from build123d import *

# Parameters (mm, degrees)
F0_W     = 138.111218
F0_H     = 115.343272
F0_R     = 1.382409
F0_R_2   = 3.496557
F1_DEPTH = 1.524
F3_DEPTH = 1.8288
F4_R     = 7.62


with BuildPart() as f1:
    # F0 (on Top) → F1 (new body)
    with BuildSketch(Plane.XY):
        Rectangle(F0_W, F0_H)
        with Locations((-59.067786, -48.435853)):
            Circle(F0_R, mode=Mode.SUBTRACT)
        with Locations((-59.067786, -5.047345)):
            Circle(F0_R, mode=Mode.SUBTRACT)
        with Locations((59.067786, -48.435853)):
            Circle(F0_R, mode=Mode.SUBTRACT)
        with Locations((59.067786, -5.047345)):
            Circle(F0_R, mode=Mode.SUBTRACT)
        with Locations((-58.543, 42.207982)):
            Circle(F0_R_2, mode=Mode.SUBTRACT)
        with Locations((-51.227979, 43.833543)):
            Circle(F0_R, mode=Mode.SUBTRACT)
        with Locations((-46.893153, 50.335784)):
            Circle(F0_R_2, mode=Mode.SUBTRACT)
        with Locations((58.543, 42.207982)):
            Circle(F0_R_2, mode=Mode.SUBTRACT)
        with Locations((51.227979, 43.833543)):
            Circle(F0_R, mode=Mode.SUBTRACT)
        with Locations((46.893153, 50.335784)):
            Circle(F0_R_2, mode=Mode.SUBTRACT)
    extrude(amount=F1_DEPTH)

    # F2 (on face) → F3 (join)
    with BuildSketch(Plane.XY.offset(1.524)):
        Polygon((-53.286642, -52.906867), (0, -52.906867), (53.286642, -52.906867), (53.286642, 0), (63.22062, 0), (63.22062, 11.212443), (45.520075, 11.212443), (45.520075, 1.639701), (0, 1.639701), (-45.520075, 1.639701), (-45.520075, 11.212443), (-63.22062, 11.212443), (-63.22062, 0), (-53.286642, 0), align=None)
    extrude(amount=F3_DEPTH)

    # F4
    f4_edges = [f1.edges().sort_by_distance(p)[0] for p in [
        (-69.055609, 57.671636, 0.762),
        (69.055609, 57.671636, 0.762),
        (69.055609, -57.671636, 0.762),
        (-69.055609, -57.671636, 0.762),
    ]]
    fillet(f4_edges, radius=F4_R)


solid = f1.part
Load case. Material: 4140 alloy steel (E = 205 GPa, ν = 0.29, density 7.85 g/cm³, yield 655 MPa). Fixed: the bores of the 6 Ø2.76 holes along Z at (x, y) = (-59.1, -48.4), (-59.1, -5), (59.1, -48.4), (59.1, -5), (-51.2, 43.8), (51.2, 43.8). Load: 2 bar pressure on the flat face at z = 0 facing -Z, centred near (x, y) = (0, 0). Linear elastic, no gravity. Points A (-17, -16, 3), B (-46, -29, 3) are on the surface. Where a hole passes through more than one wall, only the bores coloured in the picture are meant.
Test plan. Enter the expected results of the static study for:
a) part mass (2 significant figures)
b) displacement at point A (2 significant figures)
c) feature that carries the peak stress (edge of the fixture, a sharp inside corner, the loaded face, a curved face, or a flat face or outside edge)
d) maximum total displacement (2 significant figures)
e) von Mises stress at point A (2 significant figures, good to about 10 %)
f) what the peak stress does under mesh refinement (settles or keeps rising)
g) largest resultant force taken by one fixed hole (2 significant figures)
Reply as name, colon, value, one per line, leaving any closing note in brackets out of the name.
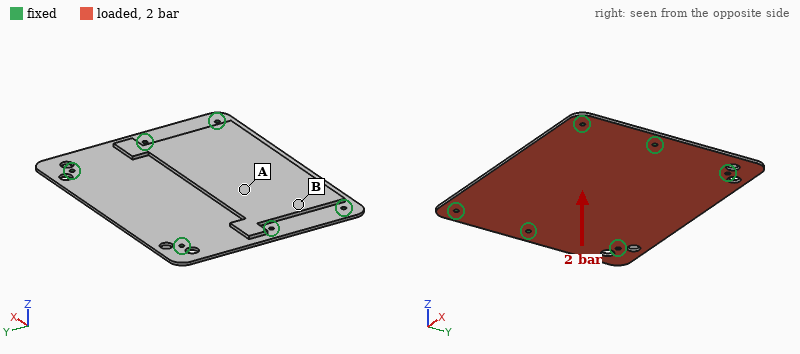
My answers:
part mass: 280 g
displacement at point A: 0.44 mm
feature that carries the peak stress: edge of the fixture
maximum total displacement: 1.1 mm
von Mises stress at point A: 150 MPa
what the peak stress does under mesh refinement: keeps rising
largest resultant force taken by one fixed hole: 2.2 kN
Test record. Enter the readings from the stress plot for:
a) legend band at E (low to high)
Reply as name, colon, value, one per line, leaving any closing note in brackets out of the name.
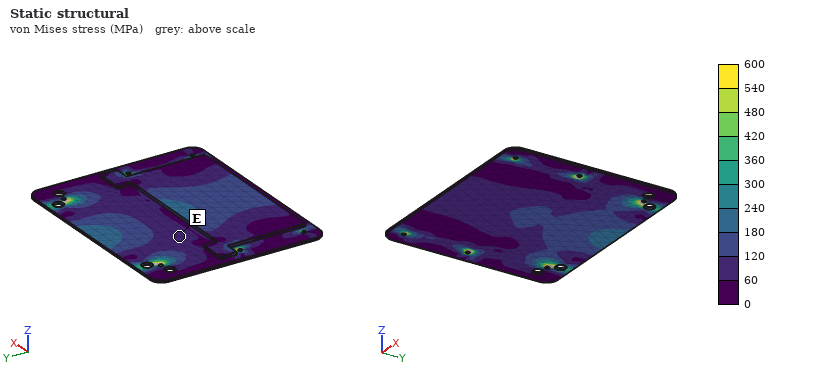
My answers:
legend band at E: 60 to 120 MPa
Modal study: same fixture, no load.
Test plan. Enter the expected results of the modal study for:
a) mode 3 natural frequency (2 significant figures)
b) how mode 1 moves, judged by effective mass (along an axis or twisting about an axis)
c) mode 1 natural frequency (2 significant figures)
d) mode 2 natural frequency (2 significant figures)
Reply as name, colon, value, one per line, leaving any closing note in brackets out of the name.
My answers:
mode 3 natural frequency: 1600 Hz
how mode 1 moves, judged by effective mass: along Z
mode 1 natural frequency: 750 Hz
mode 2 natural frequency: 950 Hz
